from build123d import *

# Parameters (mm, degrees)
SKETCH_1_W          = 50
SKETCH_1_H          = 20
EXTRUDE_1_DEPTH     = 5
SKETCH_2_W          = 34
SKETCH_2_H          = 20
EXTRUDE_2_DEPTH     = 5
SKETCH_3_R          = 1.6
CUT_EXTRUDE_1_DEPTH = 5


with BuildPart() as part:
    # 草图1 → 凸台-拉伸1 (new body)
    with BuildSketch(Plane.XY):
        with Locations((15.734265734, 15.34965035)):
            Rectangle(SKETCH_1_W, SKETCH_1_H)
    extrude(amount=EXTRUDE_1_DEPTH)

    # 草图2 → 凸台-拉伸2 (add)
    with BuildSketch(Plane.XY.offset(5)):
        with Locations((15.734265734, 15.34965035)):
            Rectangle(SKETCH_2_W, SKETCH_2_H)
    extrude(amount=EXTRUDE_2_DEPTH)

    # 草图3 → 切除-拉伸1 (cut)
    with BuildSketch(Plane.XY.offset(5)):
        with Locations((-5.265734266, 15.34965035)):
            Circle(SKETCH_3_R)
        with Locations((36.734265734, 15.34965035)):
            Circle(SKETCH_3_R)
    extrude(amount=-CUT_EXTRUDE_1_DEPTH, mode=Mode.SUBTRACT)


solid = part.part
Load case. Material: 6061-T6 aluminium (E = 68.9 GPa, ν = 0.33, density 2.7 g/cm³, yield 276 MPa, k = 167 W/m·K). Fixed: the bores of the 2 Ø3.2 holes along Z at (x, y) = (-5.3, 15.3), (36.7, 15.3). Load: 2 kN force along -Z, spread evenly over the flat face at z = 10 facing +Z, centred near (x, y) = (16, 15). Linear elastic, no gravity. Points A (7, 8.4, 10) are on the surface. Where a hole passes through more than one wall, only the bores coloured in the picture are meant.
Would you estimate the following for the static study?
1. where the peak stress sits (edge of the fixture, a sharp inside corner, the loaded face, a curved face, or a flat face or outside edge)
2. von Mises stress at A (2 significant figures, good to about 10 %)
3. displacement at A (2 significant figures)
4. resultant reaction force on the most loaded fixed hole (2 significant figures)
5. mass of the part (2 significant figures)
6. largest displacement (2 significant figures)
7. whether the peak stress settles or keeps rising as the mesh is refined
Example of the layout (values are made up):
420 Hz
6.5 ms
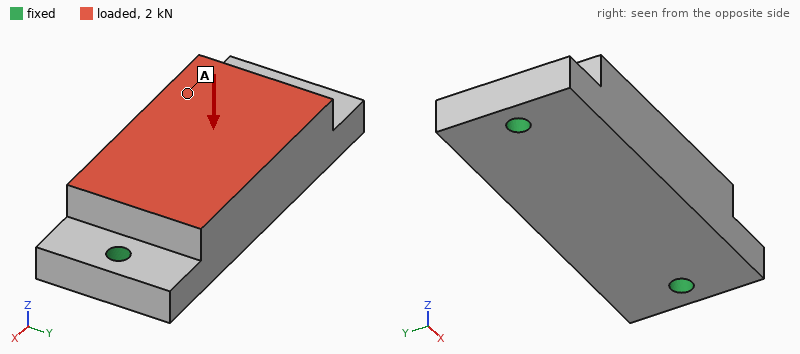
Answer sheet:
edge of the fixture
17 MPa
13 µm
1.2 kN
22 g
16 µm
keeps rising
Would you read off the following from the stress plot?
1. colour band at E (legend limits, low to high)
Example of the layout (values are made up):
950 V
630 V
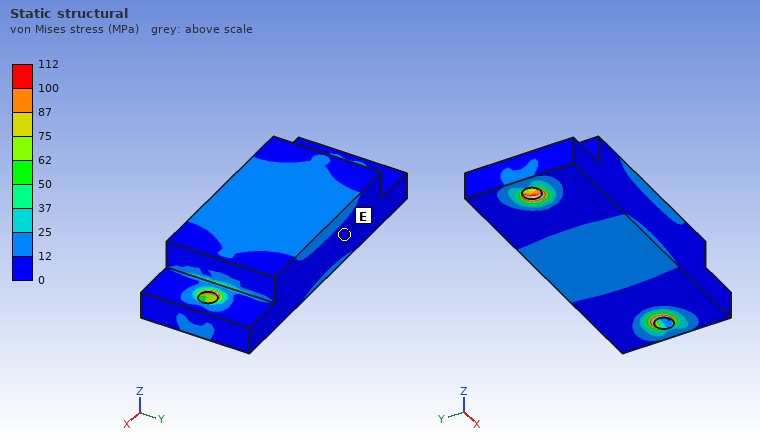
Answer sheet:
0 to 12 MPa
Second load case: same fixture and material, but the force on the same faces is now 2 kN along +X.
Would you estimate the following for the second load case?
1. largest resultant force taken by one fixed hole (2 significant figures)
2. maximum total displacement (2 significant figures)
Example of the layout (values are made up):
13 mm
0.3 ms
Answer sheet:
1.1 kN
4.3 µm
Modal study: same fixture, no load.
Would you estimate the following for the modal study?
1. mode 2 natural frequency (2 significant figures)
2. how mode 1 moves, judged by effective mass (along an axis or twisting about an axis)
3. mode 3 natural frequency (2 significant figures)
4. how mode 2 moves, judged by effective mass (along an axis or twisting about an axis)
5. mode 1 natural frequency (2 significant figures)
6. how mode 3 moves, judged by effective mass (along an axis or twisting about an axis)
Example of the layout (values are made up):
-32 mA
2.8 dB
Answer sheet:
14 kHz
along Y
21 kHz
along Z
12 kHz
along Y
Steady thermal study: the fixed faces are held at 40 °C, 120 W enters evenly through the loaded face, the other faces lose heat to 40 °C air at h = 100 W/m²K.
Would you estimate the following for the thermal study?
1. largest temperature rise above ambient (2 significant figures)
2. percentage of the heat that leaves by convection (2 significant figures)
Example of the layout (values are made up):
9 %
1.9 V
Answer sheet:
45 K
5.5 %
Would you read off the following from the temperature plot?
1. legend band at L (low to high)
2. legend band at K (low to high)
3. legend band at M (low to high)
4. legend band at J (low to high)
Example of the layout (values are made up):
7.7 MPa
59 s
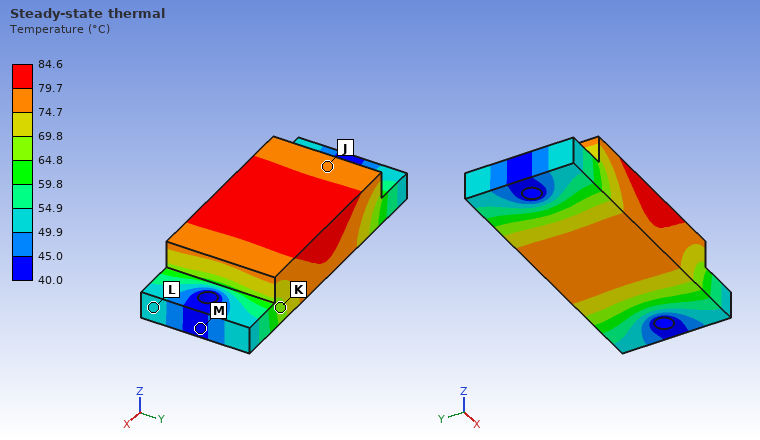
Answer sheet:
49.9 to 54.9 °C
64.8 to 69.8 °C
40.0 to 45.0 °C
74.7 to 79.7 °C
